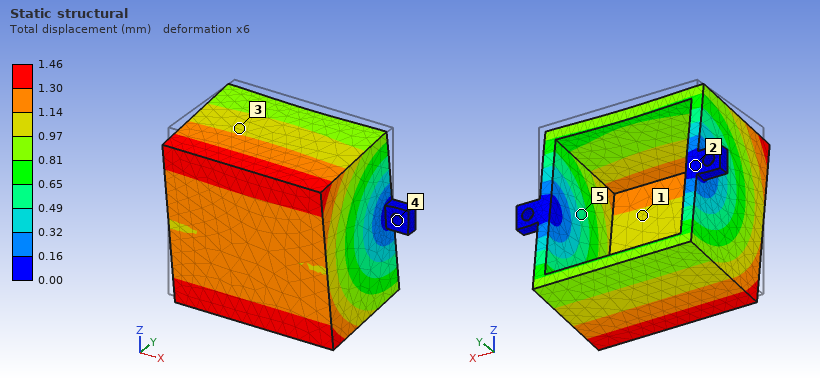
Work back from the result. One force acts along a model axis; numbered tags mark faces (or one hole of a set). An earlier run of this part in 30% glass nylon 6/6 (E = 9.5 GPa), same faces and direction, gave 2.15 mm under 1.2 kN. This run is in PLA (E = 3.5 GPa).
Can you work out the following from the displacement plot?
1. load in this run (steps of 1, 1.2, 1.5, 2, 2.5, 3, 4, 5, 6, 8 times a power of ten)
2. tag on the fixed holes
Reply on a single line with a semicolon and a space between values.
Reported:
300 N; 4
